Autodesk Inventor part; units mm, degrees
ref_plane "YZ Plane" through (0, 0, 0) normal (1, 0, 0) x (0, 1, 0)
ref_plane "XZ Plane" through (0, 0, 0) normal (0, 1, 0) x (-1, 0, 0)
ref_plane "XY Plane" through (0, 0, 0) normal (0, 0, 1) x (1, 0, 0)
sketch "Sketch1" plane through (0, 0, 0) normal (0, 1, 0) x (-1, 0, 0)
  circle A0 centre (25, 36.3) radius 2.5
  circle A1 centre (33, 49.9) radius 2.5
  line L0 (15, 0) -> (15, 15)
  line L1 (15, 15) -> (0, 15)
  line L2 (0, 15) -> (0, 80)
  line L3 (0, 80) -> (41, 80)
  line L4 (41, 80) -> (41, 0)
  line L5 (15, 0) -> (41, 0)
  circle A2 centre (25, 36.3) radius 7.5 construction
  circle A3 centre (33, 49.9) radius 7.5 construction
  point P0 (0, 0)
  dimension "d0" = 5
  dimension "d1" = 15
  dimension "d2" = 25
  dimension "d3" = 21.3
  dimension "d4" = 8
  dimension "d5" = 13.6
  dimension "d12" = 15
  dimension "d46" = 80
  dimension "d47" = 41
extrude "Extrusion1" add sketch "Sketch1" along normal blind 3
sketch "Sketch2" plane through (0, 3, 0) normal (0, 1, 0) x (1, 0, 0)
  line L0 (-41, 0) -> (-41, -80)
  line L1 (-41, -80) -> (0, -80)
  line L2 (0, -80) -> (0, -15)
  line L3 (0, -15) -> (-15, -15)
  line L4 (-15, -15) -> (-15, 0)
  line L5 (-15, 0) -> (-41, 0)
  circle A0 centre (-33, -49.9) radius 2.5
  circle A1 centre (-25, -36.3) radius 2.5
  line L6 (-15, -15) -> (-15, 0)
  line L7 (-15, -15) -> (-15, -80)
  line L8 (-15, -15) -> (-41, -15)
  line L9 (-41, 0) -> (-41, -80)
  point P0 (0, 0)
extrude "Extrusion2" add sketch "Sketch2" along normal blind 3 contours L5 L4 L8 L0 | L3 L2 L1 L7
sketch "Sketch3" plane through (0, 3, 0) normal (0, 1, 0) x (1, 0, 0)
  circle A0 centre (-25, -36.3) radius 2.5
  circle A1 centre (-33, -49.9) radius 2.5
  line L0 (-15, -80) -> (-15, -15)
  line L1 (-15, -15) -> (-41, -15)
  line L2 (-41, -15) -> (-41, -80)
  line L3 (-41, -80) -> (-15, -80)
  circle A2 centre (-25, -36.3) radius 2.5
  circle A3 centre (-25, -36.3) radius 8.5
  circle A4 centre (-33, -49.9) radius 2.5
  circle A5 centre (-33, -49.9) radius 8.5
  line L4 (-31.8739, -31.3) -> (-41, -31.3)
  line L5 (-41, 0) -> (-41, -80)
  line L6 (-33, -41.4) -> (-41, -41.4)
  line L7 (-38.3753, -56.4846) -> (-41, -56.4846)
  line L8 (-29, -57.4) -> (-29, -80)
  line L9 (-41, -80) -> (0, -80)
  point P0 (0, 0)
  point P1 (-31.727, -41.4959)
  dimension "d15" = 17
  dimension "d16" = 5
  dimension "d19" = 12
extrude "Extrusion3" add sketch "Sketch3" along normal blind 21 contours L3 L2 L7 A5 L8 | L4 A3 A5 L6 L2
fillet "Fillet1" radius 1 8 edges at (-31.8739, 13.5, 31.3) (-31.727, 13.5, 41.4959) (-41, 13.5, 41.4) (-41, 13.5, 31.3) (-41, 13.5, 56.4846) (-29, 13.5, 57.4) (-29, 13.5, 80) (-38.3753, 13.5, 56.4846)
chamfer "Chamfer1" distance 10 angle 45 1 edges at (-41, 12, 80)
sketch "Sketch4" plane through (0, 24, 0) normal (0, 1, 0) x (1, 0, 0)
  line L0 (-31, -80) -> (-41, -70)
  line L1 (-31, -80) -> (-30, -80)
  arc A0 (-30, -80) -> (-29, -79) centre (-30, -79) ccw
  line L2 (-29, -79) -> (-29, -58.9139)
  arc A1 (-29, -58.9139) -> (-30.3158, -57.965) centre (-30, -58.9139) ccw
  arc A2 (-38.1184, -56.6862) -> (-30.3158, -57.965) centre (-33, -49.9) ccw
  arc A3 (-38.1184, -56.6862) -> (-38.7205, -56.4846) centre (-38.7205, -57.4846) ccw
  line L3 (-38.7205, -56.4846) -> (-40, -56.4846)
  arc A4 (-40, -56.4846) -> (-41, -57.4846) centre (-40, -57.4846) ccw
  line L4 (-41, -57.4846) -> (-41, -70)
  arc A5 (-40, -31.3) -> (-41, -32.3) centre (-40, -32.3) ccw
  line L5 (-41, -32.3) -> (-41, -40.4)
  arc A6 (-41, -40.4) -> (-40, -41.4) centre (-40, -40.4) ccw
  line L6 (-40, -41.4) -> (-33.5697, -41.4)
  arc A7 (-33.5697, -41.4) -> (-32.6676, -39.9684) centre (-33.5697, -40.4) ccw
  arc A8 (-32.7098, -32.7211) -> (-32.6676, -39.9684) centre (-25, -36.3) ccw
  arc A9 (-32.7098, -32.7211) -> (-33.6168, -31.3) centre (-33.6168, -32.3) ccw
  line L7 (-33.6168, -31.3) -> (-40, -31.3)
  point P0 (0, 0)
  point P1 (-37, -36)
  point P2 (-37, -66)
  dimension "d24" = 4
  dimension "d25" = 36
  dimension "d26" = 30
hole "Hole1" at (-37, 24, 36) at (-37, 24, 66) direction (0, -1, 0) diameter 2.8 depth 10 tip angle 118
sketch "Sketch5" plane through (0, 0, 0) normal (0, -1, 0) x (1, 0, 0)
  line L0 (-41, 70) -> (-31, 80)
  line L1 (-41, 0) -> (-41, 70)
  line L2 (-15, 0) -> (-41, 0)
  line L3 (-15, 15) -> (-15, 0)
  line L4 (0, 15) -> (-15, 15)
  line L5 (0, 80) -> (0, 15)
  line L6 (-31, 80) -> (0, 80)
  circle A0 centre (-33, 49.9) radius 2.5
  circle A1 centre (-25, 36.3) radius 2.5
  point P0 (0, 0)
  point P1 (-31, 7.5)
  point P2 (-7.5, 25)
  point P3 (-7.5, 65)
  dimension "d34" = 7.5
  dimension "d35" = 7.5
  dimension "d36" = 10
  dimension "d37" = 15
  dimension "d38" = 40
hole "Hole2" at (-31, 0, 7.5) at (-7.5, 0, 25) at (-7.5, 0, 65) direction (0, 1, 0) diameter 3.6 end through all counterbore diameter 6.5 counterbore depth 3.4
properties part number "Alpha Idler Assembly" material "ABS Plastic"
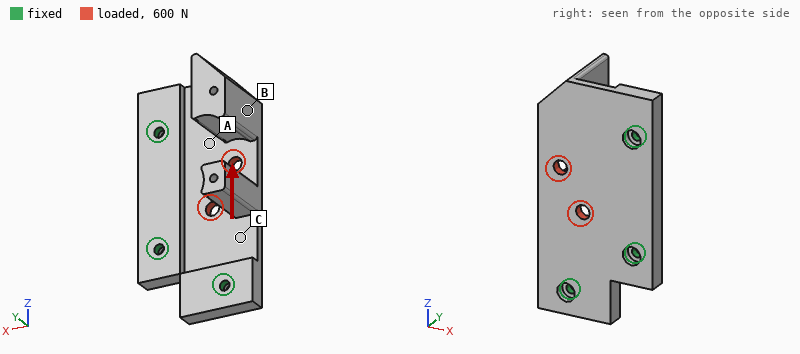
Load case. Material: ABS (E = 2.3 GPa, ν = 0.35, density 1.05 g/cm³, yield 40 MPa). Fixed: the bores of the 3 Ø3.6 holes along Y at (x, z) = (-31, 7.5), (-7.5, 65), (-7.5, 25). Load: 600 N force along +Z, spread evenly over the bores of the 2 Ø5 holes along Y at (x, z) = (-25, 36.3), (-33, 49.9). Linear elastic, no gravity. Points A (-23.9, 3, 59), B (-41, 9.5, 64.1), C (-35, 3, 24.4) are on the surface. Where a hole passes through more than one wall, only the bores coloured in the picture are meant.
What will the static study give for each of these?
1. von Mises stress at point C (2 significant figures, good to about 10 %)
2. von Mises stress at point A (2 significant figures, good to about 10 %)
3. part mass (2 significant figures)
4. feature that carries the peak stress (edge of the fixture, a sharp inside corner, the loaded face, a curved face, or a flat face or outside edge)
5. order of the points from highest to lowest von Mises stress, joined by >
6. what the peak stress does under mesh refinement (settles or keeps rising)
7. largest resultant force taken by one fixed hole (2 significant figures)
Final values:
7.0 MPa
3.8 MPa
20 g
edge of the fixture
C > A > B
keeps rising
260 N
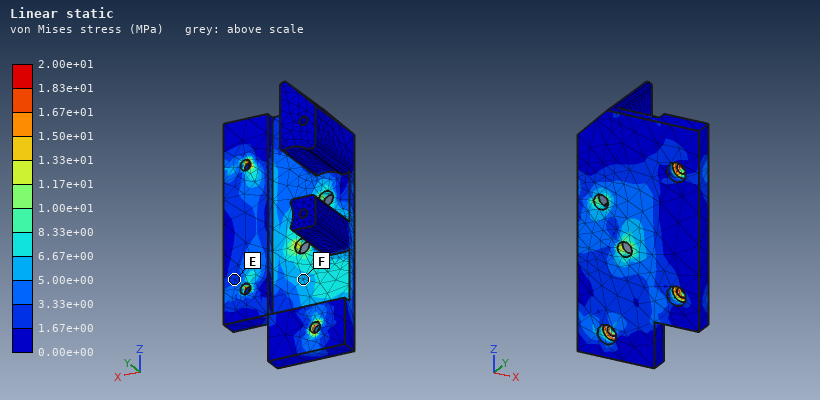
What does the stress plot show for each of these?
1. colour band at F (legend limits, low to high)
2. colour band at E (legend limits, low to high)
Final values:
5.00e+00 to 6.67e+00 MPa
1.67e+00 to 3.33e+00 MPa
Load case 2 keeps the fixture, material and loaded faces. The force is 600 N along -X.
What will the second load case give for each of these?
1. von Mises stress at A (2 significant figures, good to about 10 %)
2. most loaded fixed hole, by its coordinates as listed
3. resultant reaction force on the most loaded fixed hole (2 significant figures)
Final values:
4.9 MPa
(-7.5, 25)
290 N
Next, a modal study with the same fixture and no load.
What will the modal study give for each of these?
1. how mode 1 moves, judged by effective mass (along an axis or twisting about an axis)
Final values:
along Y
